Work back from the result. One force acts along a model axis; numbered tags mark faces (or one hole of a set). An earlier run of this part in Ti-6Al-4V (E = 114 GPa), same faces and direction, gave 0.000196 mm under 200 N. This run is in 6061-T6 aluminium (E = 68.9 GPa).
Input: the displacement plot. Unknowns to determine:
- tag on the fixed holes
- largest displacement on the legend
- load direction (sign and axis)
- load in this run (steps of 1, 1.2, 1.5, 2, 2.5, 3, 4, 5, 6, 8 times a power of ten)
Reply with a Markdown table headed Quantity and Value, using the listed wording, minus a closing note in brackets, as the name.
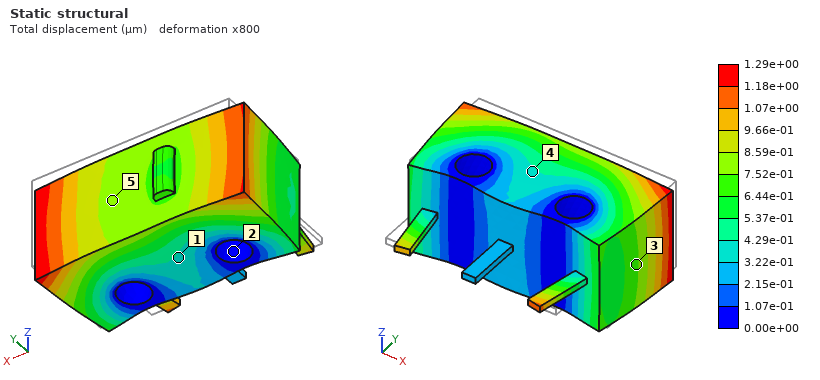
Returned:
| Quantity | Value |
|---|---|
| tag on the fixed holes | 2 |
| largest displacement on the legend | 1.29e+00 µm |
| load direction | -Y |
| load in this run | 800 N |
